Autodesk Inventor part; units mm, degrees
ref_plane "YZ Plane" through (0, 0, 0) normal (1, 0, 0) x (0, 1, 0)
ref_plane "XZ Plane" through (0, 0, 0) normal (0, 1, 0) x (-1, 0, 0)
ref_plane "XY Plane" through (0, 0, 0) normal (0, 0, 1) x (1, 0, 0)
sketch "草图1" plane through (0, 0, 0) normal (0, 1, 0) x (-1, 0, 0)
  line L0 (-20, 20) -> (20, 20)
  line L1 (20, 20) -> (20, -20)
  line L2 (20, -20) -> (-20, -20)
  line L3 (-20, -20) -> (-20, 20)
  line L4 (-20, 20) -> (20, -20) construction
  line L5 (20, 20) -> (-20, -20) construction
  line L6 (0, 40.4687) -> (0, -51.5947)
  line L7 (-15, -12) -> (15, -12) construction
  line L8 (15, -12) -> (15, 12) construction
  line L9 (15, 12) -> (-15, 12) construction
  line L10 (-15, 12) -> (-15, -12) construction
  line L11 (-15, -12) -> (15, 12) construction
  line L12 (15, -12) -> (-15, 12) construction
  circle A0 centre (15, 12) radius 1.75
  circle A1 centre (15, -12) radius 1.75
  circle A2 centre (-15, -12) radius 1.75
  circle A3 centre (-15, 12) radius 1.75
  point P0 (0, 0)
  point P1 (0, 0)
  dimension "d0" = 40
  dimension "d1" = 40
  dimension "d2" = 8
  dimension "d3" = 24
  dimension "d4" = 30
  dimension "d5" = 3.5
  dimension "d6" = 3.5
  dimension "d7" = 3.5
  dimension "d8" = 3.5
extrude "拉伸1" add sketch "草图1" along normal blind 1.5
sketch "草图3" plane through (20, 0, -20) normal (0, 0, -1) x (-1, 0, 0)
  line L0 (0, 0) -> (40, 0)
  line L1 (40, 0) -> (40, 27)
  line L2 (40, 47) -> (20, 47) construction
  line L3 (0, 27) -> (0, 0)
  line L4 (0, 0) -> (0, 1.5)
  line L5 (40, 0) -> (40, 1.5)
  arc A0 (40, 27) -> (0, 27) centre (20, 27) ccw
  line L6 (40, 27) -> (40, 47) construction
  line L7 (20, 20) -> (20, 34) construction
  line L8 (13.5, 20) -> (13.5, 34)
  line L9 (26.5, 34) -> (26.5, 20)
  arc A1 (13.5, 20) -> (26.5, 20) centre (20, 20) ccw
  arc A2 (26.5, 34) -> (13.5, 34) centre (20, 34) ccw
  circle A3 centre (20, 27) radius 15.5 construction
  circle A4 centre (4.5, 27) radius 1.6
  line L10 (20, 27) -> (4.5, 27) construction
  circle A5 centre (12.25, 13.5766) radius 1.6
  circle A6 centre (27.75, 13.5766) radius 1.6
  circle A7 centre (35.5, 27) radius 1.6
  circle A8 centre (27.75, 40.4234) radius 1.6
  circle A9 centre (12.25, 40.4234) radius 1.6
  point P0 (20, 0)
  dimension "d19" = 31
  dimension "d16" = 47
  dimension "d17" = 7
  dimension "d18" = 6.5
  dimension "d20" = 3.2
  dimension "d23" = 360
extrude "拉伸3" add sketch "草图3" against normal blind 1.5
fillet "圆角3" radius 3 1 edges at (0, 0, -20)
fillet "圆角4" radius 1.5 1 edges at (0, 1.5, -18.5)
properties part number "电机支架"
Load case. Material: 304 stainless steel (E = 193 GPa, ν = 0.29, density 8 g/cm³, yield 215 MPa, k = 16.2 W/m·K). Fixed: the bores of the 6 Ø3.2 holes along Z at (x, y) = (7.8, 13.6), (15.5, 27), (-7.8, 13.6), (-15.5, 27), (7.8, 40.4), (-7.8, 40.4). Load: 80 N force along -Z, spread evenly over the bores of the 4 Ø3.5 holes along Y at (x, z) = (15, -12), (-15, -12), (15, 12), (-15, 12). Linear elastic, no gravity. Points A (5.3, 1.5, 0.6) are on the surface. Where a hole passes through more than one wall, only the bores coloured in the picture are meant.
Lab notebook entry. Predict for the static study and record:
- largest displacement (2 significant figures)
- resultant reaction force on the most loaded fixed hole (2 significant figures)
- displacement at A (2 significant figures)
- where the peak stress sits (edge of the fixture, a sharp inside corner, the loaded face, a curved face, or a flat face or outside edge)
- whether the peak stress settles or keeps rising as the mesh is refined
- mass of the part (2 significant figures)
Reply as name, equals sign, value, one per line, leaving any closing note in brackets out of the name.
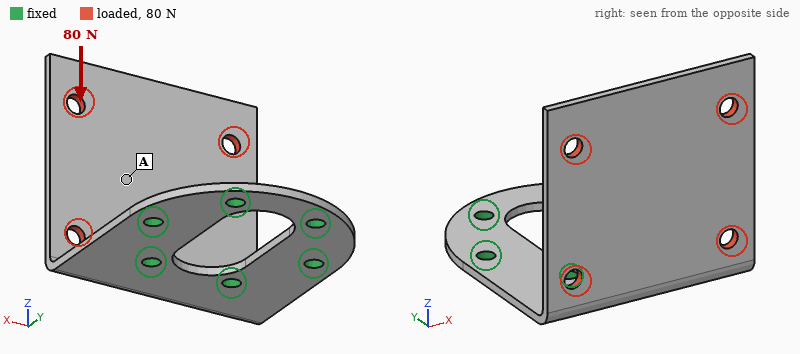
largest displacement = 0.12 mm
resultant reaction force on the most loaded fixed hole = 48 N
displacement at A = 0.063 mm
where the peak stress sits = edge of the fixture
whether the peak stress settles or keeps rising as the mesh is refined = keeps rising
mass of the part = 34 g
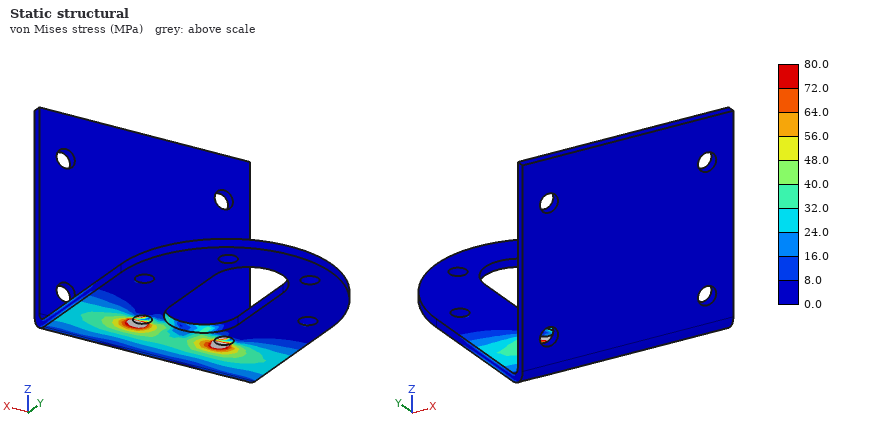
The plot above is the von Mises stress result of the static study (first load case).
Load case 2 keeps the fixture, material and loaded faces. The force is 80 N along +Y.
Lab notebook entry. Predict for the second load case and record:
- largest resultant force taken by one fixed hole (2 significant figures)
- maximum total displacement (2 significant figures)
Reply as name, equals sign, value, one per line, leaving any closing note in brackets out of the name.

largest resultant force taken by one fixed hole = 36 N
maximum total displacement = 0.60 mm
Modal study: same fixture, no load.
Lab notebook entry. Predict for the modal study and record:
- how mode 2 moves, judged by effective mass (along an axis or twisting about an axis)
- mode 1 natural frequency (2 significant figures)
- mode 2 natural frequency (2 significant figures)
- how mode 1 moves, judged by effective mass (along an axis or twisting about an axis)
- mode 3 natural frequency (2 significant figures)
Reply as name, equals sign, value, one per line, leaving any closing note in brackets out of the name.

how mode 2 moves, judged by effective mass = along X
mode 1 natural frequency = 520 Hz
mode 2 natural frequency = 1200 Hz
how mode 1 moves, judged by effective mass = along Y
mode 3 natural frequency = 1900 Hz
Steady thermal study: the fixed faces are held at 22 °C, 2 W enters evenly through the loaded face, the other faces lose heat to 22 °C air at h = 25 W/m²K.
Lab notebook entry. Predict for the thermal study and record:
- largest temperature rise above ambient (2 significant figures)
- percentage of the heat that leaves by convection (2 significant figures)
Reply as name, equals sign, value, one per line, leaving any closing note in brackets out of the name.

largest temperature rise above ambient = 25 K
percentage of the heat that leaves by convection = 72 %
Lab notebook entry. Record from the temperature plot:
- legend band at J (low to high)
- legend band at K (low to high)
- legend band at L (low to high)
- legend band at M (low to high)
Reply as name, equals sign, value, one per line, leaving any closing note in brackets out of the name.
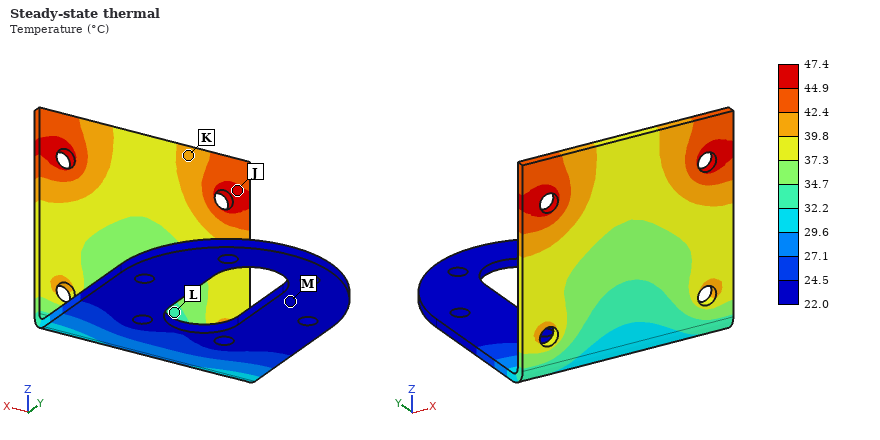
legend band at J = 44.9 to 47.4 °C
legend band at K = 39.8 to 42.4 °C
legend band at L = 32.2 to 34.7 °C
legend band at M = 22.0 to 24.5 °C
